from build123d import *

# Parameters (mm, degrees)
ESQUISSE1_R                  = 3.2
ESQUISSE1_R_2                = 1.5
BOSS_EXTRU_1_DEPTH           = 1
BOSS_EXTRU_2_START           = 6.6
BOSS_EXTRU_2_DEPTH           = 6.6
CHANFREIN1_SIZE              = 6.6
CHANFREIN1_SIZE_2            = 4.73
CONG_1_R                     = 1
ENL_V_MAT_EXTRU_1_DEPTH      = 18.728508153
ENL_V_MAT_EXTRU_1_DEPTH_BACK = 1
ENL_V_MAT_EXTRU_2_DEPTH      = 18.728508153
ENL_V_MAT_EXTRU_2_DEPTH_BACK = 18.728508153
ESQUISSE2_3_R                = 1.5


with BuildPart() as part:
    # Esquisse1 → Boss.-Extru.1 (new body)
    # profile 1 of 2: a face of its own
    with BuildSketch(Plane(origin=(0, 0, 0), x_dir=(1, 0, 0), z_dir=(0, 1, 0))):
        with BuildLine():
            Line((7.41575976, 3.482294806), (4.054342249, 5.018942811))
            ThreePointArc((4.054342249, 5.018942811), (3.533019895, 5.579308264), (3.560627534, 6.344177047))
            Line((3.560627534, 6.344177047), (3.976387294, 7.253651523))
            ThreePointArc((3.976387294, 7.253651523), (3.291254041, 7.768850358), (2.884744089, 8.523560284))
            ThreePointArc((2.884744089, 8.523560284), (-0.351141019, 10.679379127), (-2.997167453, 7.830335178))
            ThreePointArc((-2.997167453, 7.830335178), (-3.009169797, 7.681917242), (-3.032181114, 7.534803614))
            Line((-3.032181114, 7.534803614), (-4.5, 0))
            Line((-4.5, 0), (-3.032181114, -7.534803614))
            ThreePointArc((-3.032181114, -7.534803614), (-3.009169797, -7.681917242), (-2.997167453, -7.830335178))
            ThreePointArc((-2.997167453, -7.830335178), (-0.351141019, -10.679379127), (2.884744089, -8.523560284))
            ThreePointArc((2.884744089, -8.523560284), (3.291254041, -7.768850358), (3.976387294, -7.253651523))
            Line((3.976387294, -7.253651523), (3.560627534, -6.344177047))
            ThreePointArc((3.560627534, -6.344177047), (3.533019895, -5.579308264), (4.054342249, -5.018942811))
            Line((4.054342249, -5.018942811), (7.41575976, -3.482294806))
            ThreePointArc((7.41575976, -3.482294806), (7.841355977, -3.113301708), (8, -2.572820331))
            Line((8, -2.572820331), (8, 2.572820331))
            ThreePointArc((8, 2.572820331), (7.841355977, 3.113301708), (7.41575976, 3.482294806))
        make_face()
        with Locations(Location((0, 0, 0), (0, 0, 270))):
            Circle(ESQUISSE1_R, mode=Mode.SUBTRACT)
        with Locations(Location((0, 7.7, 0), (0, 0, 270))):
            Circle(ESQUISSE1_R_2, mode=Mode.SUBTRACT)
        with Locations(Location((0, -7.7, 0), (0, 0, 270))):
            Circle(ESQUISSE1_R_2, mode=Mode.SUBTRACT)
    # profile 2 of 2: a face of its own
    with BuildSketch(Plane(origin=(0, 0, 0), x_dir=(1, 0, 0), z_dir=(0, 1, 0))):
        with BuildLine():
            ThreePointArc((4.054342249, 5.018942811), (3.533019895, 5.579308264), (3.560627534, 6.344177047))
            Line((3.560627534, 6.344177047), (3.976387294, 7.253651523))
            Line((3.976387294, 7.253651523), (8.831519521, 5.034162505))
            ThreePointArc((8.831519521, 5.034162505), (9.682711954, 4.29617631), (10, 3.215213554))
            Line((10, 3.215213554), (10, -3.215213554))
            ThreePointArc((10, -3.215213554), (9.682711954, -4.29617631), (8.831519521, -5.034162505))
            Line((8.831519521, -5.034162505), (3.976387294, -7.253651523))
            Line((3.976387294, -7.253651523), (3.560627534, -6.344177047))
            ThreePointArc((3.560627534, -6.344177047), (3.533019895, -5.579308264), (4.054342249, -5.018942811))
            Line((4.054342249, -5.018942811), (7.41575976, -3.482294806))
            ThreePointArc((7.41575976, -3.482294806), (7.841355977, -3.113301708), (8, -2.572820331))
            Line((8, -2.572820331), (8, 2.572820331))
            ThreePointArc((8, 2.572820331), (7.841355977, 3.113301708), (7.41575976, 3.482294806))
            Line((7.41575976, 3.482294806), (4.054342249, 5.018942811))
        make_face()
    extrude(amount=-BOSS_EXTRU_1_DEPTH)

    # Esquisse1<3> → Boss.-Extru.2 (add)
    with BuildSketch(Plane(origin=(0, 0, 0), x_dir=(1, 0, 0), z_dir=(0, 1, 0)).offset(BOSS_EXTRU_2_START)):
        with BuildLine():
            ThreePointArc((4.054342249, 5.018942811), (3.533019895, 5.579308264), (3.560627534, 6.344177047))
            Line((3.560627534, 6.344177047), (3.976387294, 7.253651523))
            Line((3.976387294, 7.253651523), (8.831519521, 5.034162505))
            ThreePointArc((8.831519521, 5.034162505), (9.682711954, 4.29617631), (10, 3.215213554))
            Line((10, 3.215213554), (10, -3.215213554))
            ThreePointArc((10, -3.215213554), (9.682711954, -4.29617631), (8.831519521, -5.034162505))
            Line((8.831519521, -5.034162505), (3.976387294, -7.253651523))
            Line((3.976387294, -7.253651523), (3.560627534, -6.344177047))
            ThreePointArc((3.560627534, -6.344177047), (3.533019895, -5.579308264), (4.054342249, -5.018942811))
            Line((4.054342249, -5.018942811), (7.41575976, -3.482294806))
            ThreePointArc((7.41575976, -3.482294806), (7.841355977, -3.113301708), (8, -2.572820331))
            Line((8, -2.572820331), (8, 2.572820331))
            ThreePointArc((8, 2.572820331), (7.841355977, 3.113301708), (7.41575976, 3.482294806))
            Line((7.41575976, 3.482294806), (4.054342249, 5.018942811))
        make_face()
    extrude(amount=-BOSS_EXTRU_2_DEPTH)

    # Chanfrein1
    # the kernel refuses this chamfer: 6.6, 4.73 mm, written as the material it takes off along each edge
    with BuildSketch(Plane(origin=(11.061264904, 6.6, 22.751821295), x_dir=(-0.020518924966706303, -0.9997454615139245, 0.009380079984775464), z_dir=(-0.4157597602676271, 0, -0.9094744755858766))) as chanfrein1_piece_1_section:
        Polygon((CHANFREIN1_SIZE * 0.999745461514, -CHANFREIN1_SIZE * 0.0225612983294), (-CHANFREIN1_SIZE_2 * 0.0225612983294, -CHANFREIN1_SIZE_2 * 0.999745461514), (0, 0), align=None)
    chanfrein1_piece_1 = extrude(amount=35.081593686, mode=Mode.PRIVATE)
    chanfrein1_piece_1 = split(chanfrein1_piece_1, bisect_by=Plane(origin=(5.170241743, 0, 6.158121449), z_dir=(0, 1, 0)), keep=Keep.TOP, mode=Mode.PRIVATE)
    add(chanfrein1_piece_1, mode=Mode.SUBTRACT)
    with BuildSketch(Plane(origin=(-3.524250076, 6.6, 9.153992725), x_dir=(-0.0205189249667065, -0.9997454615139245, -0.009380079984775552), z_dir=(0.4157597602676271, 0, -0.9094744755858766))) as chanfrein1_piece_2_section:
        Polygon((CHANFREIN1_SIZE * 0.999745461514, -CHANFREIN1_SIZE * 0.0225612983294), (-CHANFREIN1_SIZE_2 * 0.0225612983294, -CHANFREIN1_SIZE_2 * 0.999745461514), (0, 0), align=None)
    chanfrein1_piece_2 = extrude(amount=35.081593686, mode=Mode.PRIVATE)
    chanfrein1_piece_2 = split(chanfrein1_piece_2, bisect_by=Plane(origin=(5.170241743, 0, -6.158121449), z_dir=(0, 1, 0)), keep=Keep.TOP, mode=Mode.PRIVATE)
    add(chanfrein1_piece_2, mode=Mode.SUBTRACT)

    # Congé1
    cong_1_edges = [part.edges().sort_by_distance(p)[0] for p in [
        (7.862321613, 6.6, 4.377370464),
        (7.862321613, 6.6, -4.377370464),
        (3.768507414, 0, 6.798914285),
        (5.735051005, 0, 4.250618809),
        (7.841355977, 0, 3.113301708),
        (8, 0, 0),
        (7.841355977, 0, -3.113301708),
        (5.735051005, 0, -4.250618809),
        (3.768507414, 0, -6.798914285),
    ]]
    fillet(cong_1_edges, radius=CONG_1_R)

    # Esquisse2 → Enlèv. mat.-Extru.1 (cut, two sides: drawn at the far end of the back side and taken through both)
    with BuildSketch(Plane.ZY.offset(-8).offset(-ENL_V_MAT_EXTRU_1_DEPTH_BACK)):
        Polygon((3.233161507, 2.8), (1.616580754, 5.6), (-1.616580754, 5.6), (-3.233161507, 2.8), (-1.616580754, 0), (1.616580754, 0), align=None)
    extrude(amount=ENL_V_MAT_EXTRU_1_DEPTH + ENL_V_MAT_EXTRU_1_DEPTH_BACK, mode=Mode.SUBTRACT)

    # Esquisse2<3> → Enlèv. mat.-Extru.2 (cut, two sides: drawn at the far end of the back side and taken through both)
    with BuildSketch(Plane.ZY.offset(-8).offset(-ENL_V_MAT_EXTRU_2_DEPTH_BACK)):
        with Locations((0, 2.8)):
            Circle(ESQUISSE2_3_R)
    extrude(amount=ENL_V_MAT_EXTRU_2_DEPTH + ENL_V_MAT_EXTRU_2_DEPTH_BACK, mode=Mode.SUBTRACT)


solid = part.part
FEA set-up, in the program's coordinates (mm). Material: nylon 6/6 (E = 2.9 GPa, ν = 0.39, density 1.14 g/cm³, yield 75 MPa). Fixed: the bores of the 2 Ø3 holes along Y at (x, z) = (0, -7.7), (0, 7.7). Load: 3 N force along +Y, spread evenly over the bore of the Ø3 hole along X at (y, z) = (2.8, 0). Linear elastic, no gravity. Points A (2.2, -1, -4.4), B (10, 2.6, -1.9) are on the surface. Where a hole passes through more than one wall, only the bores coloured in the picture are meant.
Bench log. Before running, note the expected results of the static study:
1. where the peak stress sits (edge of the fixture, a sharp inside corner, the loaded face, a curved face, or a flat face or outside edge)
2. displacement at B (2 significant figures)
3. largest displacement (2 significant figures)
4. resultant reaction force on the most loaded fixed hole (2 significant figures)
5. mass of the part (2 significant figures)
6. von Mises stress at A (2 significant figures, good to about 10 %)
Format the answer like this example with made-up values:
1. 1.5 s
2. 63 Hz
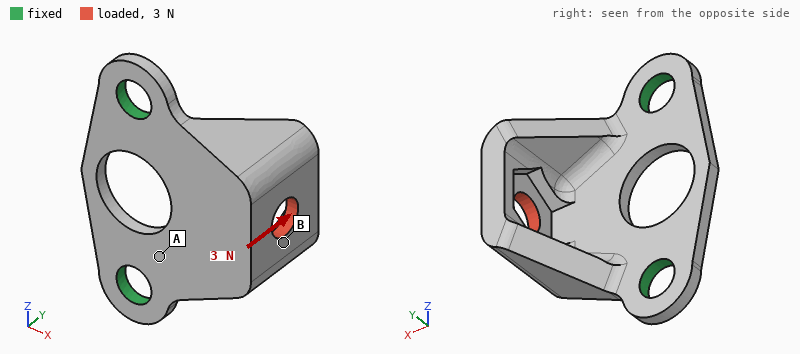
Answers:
1. a flat face or outside edge
2. 0.21 mm
3. 0.27 mm
4. 1.5 N
5. 0.38 g
6. 8.4 MPa
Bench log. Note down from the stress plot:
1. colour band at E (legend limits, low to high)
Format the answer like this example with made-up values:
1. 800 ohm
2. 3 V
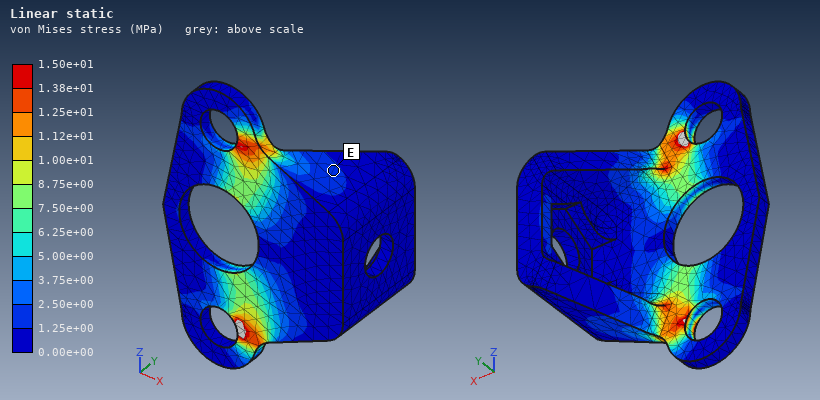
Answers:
1. 1.25e+00 to 2.50e+00 MPa
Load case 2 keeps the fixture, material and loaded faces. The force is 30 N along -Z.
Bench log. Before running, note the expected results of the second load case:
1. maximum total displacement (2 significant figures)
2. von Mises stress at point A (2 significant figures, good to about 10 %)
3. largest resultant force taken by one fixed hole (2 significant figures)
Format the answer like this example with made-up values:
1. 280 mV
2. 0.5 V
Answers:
1. 0.12 mm
2. 3.0 MPa
3. 23 N
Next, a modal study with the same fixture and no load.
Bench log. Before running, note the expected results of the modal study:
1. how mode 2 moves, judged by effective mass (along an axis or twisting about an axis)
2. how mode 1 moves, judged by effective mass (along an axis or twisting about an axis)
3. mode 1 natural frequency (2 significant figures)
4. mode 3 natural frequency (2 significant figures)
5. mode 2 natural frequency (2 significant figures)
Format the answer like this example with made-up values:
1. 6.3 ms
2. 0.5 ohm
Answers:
1. along Z
2. along Y
3. 1400 Hz
4. 9700 Hz
5. 5600 Hz
